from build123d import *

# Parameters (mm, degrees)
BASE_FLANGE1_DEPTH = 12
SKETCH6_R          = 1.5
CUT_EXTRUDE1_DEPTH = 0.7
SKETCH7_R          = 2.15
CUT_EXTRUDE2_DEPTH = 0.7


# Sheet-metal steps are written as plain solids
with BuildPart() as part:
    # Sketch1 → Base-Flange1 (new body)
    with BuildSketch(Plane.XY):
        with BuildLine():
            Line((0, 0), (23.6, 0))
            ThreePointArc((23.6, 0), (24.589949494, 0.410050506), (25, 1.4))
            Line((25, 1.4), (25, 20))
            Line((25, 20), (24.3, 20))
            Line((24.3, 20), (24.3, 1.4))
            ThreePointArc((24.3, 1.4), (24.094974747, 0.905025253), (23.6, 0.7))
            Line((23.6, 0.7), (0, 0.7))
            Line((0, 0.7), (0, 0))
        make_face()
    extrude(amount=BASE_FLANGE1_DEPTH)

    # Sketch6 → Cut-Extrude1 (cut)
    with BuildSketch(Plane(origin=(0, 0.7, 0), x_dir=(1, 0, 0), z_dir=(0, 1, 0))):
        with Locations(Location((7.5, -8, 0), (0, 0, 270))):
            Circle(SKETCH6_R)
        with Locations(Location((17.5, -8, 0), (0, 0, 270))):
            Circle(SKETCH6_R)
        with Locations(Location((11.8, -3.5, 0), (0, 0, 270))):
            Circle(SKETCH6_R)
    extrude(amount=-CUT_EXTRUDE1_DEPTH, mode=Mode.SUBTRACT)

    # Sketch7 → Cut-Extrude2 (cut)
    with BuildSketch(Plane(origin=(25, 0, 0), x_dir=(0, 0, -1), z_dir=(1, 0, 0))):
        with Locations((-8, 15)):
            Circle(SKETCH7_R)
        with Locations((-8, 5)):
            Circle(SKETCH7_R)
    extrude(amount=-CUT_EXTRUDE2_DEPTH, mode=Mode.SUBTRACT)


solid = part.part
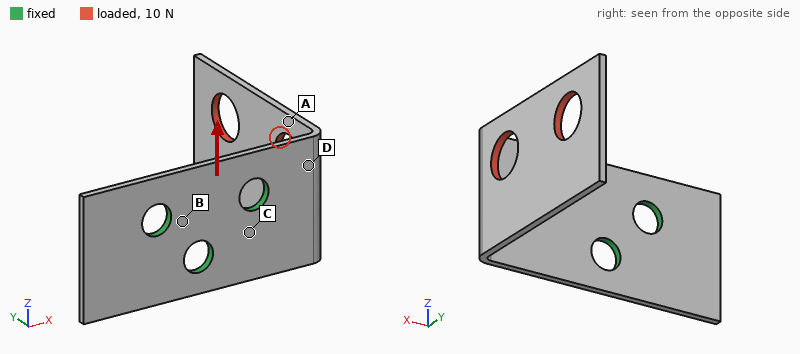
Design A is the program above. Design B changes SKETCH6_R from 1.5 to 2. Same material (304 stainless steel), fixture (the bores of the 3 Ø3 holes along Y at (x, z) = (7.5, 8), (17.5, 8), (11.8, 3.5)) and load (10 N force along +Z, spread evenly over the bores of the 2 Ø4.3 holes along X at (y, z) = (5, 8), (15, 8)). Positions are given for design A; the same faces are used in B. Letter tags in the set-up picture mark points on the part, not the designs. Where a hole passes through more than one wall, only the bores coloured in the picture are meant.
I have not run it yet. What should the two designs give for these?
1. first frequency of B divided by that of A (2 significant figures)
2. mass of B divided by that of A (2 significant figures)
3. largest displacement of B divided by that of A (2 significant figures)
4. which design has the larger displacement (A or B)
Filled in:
1.0
0.97
0.86
A
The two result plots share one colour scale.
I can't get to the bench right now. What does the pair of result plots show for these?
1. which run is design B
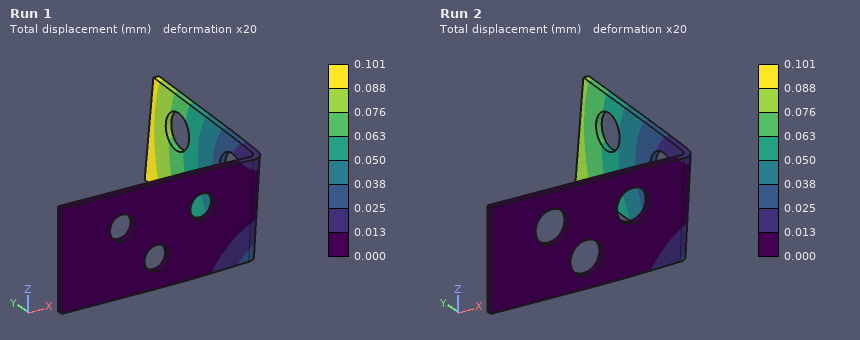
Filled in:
Run 2
